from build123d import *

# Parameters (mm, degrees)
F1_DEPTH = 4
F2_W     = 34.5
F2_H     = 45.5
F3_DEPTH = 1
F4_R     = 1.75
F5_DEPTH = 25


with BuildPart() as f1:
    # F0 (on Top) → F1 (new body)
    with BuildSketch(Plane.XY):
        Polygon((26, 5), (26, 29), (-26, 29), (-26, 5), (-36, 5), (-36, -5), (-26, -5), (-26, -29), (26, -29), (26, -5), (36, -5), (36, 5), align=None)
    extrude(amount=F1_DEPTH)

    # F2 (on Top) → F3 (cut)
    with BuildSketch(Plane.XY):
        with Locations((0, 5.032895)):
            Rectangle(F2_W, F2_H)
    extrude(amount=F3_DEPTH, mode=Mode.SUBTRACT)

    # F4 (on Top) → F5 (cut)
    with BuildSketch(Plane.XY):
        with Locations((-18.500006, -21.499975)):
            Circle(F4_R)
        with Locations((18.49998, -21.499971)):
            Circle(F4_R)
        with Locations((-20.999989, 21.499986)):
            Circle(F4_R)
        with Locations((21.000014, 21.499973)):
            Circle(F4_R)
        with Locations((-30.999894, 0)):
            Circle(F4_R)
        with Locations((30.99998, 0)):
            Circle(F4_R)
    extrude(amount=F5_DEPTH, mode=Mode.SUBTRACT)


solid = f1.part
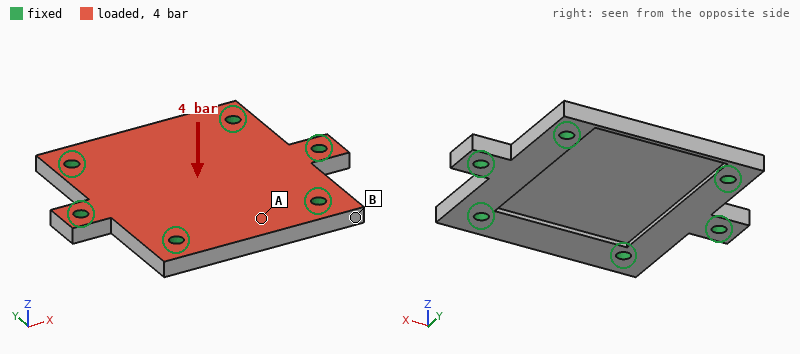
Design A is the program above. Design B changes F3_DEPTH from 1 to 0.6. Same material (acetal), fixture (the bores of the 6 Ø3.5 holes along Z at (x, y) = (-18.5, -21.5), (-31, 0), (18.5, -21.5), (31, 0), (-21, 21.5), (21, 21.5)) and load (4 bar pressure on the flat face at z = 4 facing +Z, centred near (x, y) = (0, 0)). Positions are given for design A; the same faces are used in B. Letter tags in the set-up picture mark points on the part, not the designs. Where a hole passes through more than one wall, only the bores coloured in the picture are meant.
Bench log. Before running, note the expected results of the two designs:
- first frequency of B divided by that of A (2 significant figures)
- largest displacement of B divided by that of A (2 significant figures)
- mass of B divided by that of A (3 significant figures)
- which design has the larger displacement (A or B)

1.0
0.83
1.06
A
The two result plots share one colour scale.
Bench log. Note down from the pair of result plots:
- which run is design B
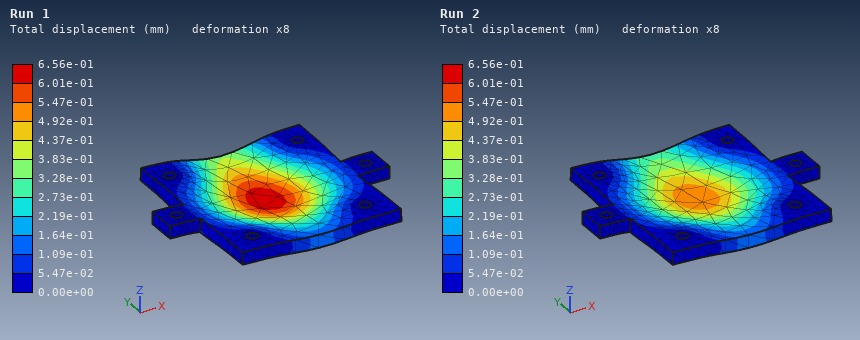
Run 2
